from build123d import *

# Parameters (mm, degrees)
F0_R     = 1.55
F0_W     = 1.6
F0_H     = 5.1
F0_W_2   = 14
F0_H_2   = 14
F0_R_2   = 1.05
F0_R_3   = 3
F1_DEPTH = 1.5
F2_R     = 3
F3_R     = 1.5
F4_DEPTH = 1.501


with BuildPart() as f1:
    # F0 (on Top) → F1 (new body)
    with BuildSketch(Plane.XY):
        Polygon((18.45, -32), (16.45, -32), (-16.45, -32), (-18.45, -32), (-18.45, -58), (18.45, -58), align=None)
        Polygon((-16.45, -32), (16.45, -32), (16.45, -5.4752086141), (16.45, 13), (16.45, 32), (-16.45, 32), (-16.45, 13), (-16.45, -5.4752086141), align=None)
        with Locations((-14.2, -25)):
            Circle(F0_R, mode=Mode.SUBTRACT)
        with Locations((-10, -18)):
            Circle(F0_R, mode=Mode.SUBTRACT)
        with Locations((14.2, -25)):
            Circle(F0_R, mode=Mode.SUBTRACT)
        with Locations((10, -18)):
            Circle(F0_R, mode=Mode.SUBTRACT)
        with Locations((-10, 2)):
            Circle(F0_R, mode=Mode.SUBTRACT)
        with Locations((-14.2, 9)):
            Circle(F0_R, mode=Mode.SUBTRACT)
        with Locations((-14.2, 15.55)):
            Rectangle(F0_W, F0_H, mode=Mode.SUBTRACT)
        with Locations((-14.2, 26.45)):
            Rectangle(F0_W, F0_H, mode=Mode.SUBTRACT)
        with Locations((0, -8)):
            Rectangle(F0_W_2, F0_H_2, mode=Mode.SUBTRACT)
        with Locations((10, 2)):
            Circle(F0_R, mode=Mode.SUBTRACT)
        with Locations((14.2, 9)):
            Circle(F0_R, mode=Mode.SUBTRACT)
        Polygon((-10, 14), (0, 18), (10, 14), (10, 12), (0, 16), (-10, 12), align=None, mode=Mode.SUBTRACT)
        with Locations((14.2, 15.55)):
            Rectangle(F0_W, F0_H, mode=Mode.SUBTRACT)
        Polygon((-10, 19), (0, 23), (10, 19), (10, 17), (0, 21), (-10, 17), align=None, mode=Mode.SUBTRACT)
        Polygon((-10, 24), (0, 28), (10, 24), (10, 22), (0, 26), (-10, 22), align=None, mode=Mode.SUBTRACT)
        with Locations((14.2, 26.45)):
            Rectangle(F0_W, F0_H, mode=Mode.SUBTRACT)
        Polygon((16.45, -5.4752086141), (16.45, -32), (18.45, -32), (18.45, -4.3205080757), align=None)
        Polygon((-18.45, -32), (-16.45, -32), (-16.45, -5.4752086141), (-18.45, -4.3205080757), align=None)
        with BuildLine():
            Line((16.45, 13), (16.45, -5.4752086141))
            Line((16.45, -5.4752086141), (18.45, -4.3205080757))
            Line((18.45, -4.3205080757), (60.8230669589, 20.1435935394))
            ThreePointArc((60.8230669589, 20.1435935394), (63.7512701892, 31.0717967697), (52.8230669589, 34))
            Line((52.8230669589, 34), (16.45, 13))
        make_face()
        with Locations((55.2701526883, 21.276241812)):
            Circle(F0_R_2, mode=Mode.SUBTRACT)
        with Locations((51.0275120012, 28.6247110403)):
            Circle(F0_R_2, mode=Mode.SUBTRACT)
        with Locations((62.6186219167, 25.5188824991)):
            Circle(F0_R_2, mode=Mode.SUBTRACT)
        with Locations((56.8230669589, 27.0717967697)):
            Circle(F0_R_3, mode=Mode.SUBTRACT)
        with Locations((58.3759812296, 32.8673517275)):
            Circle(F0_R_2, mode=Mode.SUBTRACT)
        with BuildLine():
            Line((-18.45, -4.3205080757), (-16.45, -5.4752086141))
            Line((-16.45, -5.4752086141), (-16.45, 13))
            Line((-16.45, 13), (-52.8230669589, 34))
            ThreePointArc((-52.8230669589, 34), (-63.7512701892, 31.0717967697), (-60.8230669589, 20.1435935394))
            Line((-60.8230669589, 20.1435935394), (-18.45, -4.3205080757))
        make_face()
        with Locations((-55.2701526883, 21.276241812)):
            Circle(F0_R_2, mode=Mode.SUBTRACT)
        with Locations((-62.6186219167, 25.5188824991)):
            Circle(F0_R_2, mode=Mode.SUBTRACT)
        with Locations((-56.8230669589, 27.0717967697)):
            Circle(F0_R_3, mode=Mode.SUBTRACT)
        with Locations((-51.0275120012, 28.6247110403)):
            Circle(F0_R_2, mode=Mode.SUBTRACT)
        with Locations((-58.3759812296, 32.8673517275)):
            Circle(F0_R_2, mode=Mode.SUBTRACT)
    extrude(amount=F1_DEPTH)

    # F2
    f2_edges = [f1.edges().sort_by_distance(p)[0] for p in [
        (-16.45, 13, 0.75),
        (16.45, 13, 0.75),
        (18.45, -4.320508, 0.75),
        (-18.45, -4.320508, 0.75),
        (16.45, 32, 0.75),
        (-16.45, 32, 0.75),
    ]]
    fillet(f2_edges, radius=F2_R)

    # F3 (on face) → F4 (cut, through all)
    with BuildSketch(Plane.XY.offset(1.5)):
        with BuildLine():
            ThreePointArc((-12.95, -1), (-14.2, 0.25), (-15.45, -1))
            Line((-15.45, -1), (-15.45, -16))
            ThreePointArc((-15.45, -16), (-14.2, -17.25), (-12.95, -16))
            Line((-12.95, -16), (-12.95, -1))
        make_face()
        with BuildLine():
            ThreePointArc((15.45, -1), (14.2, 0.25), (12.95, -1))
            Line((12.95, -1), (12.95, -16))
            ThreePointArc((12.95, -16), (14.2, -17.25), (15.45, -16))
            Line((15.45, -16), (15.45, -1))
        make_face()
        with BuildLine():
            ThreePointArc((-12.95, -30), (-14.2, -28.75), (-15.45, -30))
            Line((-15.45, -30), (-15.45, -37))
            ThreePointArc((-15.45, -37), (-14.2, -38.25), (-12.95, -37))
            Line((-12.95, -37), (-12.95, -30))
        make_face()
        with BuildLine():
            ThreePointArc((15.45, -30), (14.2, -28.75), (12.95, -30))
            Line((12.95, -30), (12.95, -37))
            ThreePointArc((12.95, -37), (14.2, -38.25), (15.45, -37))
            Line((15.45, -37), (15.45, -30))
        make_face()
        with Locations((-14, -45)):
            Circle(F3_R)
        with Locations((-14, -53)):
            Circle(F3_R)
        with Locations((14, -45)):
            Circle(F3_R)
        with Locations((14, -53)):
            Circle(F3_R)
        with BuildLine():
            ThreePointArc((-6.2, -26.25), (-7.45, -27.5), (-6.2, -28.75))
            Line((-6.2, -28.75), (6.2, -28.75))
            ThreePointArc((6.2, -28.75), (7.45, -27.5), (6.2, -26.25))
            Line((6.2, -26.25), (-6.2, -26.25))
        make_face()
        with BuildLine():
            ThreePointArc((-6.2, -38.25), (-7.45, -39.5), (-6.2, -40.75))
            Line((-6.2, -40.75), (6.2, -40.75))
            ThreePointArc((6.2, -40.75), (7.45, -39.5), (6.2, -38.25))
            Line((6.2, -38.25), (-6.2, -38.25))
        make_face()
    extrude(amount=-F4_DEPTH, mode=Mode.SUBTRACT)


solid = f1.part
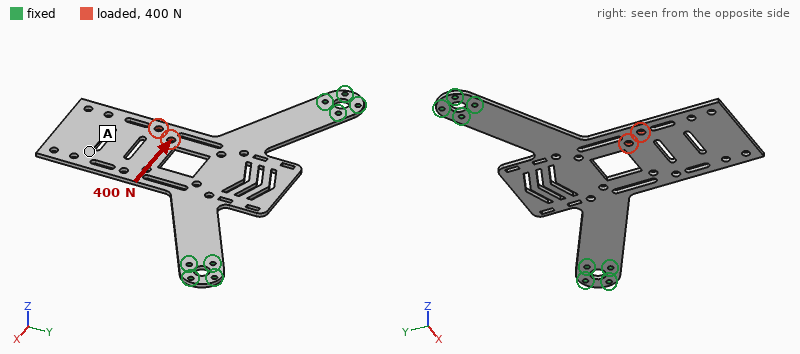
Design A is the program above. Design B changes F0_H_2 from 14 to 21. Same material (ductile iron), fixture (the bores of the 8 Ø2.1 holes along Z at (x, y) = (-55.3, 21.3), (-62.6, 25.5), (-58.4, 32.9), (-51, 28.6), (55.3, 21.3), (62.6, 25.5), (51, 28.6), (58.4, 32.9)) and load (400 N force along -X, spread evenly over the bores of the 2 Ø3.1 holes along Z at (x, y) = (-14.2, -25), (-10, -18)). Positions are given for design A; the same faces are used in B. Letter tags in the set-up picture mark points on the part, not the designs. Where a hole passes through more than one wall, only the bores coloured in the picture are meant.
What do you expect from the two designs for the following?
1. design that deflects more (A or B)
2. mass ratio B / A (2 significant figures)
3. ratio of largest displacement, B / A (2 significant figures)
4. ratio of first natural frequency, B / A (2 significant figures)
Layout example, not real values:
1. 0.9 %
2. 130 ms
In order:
1. B
2. 0.98
3. 1.1
4. 0.99
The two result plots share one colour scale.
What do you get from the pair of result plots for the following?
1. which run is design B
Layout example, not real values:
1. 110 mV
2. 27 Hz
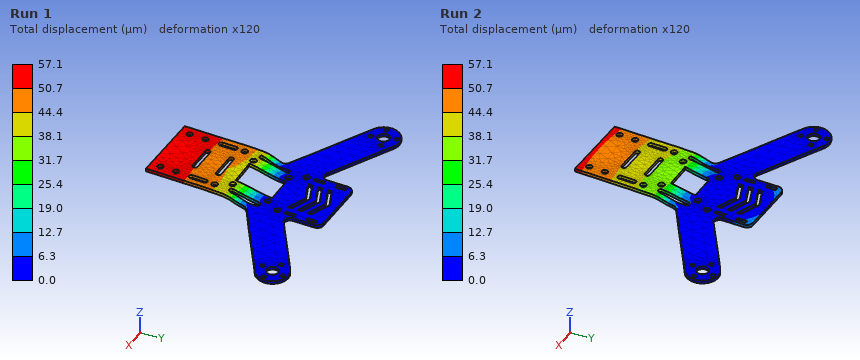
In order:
1. Run 1
